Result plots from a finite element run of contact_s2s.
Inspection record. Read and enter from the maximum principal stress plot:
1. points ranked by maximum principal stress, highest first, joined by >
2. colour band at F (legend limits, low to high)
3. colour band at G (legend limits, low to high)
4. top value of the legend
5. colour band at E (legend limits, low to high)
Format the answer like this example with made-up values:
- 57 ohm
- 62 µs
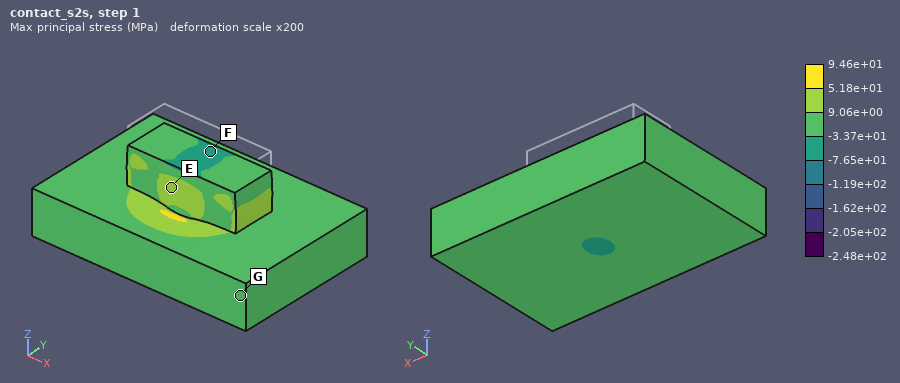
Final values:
- E > G > F
- -7.65e+01 to -3.37e+01 MPa
- -3.37e+01 to 9.06e+00 MPa
- 9.46e+01 MPa
- 9.06e+00 to 5.18e+01 MPa
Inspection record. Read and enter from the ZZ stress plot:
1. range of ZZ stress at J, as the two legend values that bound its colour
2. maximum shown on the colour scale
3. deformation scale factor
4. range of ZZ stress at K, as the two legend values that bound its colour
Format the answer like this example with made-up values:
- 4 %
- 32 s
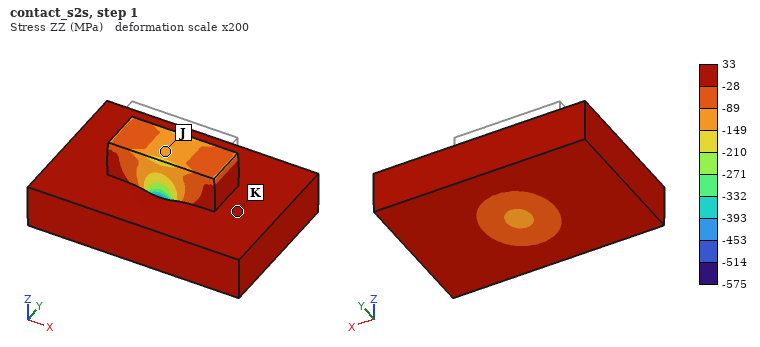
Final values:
- -149 to -89 MPa
- 33 MPa
- 200
- -28 to 33 MPa
